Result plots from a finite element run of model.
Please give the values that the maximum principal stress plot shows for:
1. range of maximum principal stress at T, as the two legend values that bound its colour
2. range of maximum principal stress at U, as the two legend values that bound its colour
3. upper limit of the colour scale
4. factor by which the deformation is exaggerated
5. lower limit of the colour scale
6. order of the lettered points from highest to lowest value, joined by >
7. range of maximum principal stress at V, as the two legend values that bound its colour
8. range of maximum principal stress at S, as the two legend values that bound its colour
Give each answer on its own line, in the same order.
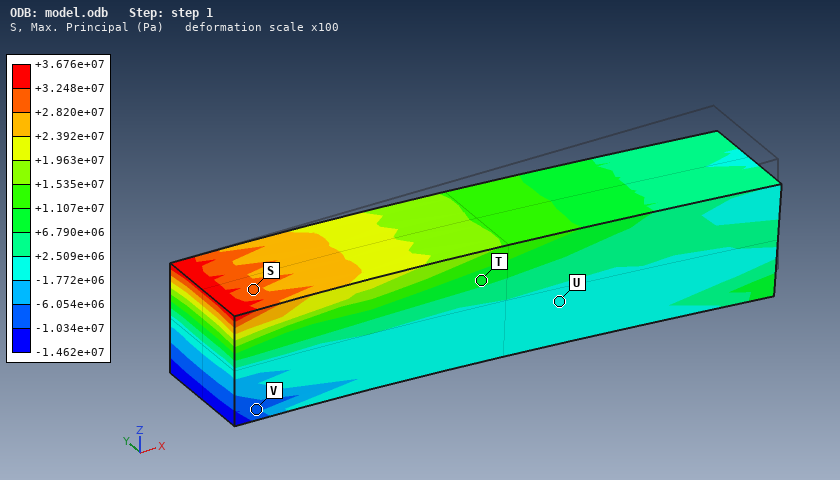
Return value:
+6.790e+06 to +1.107e+07 Pa
-1.772e+06 to +2.509e+06 Pa
+3.676e+07 Pa
100
-1.462e+07 Pa
S > T > U > V
-1.034e+07 to -6.054e+06 Pa
+2.820e+07 to +3.248e+07 Pa
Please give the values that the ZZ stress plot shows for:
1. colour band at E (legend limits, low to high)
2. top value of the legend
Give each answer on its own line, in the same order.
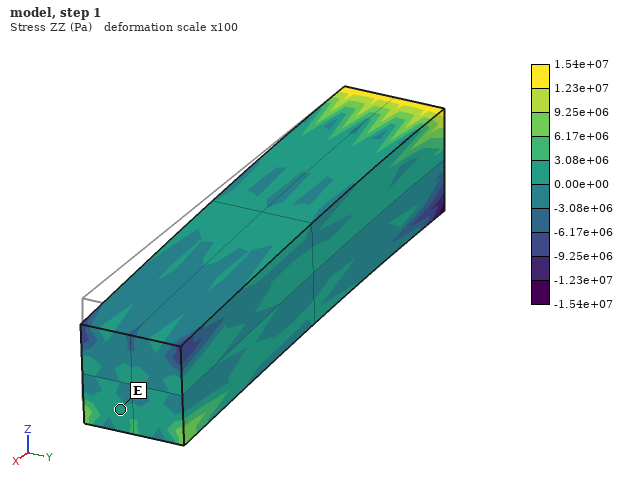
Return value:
0.00e+00 to 3.08e+06 Pa
1.54e+07 Pa
